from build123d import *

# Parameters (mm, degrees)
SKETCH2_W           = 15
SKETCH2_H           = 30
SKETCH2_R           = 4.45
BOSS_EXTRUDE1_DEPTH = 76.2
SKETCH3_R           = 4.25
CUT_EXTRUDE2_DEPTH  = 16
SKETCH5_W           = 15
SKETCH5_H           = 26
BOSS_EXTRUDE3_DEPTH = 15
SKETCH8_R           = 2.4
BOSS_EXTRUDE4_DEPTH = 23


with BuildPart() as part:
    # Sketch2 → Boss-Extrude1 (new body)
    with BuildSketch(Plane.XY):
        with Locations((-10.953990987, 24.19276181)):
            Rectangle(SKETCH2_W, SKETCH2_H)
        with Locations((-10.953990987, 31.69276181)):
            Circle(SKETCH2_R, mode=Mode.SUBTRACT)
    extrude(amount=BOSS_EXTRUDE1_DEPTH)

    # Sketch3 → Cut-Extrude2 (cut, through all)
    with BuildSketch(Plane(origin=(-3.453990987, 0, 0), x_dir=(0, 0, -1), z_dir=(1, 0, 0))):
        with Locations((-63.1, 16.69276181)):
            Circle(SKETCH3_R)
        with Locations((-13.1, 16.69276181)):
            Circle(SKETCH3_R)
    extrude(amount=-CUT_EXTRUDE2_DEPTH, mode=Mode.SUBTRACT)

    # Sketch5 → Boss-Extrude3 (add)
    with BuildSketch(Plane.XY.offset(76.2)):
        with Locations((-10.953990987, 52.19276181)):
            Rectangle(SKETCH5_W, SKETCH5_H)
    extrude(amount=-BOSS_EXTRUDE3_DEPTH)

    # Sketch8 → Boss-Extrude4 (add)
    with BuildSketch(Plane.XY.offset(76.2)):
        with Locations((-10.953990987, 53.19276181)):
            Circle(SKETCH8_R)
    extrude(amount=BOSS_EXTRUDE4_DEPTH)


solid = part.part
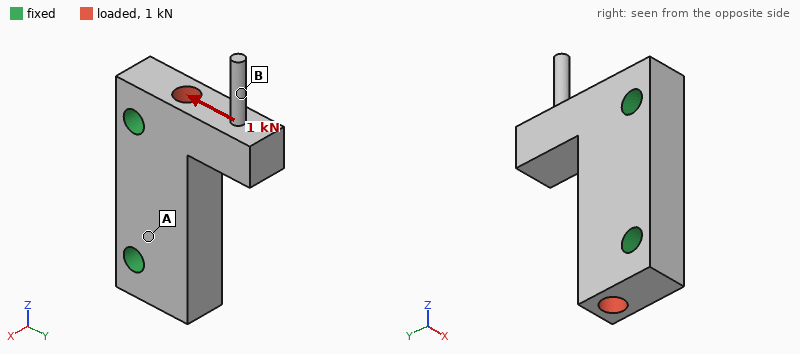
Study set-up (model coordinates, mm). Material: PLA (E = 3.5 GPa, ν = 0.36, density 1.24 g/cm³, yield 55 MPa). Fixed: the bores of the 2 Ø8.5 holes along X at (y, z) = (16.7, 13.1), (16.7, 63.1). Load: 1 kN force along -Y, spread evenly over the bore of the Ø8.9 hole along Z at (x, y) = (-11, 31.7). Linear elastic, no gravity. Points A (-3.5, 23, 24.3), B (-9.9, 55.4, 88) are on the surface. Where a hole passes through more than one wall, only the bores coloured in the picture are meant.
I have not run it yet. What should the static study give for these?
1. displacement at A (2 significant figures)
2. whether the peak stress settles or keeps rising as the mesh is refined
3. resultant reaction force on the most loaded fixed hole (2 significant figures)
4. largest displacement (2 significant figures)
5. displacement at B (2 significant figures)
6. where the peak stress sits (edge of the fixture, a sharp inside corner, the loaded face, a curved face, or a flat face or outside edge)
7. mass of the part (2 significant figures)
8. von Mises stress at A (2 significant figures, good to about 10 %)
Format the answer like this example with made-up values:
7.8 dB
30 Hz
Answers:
8.5 µm
keeps rising
510 N
18 µm
6.2 µm
edge of the fixture
42 g
1.5 MPa
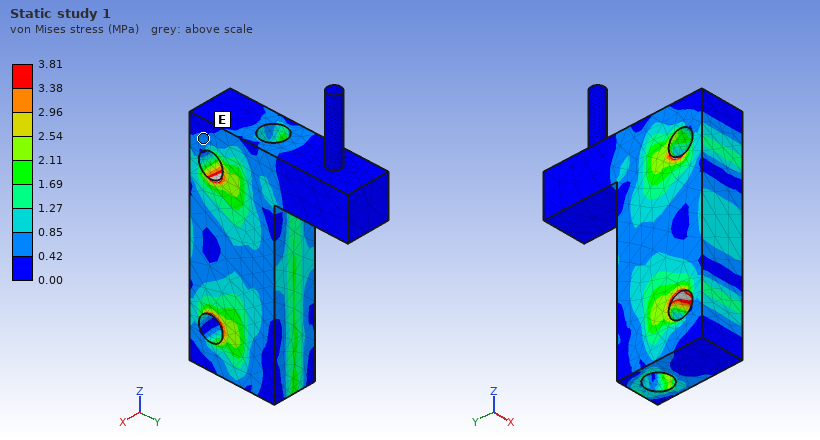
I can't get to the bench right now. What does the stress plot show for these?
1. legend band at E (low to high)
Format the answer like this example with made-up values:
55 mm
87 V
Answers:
0.42 to 0.85 MPa
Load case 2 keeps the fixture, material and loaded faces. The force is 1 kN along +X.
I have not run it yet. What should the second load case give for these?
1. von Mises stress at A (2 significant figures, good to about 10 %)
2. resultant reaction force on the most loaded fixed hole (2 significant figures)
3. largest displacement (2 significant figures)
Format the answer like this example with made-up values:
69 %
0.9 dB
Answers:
3.1 MPa
500 N
0.13 mm
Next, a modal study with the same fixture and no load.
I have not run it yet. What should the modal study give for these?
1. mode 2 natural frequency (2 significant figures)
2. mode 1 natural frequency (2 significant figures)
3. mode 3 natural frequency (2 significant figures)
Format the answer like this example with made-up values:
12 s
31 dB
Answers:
1800 Hz
1700 Hz
2100 Hz
